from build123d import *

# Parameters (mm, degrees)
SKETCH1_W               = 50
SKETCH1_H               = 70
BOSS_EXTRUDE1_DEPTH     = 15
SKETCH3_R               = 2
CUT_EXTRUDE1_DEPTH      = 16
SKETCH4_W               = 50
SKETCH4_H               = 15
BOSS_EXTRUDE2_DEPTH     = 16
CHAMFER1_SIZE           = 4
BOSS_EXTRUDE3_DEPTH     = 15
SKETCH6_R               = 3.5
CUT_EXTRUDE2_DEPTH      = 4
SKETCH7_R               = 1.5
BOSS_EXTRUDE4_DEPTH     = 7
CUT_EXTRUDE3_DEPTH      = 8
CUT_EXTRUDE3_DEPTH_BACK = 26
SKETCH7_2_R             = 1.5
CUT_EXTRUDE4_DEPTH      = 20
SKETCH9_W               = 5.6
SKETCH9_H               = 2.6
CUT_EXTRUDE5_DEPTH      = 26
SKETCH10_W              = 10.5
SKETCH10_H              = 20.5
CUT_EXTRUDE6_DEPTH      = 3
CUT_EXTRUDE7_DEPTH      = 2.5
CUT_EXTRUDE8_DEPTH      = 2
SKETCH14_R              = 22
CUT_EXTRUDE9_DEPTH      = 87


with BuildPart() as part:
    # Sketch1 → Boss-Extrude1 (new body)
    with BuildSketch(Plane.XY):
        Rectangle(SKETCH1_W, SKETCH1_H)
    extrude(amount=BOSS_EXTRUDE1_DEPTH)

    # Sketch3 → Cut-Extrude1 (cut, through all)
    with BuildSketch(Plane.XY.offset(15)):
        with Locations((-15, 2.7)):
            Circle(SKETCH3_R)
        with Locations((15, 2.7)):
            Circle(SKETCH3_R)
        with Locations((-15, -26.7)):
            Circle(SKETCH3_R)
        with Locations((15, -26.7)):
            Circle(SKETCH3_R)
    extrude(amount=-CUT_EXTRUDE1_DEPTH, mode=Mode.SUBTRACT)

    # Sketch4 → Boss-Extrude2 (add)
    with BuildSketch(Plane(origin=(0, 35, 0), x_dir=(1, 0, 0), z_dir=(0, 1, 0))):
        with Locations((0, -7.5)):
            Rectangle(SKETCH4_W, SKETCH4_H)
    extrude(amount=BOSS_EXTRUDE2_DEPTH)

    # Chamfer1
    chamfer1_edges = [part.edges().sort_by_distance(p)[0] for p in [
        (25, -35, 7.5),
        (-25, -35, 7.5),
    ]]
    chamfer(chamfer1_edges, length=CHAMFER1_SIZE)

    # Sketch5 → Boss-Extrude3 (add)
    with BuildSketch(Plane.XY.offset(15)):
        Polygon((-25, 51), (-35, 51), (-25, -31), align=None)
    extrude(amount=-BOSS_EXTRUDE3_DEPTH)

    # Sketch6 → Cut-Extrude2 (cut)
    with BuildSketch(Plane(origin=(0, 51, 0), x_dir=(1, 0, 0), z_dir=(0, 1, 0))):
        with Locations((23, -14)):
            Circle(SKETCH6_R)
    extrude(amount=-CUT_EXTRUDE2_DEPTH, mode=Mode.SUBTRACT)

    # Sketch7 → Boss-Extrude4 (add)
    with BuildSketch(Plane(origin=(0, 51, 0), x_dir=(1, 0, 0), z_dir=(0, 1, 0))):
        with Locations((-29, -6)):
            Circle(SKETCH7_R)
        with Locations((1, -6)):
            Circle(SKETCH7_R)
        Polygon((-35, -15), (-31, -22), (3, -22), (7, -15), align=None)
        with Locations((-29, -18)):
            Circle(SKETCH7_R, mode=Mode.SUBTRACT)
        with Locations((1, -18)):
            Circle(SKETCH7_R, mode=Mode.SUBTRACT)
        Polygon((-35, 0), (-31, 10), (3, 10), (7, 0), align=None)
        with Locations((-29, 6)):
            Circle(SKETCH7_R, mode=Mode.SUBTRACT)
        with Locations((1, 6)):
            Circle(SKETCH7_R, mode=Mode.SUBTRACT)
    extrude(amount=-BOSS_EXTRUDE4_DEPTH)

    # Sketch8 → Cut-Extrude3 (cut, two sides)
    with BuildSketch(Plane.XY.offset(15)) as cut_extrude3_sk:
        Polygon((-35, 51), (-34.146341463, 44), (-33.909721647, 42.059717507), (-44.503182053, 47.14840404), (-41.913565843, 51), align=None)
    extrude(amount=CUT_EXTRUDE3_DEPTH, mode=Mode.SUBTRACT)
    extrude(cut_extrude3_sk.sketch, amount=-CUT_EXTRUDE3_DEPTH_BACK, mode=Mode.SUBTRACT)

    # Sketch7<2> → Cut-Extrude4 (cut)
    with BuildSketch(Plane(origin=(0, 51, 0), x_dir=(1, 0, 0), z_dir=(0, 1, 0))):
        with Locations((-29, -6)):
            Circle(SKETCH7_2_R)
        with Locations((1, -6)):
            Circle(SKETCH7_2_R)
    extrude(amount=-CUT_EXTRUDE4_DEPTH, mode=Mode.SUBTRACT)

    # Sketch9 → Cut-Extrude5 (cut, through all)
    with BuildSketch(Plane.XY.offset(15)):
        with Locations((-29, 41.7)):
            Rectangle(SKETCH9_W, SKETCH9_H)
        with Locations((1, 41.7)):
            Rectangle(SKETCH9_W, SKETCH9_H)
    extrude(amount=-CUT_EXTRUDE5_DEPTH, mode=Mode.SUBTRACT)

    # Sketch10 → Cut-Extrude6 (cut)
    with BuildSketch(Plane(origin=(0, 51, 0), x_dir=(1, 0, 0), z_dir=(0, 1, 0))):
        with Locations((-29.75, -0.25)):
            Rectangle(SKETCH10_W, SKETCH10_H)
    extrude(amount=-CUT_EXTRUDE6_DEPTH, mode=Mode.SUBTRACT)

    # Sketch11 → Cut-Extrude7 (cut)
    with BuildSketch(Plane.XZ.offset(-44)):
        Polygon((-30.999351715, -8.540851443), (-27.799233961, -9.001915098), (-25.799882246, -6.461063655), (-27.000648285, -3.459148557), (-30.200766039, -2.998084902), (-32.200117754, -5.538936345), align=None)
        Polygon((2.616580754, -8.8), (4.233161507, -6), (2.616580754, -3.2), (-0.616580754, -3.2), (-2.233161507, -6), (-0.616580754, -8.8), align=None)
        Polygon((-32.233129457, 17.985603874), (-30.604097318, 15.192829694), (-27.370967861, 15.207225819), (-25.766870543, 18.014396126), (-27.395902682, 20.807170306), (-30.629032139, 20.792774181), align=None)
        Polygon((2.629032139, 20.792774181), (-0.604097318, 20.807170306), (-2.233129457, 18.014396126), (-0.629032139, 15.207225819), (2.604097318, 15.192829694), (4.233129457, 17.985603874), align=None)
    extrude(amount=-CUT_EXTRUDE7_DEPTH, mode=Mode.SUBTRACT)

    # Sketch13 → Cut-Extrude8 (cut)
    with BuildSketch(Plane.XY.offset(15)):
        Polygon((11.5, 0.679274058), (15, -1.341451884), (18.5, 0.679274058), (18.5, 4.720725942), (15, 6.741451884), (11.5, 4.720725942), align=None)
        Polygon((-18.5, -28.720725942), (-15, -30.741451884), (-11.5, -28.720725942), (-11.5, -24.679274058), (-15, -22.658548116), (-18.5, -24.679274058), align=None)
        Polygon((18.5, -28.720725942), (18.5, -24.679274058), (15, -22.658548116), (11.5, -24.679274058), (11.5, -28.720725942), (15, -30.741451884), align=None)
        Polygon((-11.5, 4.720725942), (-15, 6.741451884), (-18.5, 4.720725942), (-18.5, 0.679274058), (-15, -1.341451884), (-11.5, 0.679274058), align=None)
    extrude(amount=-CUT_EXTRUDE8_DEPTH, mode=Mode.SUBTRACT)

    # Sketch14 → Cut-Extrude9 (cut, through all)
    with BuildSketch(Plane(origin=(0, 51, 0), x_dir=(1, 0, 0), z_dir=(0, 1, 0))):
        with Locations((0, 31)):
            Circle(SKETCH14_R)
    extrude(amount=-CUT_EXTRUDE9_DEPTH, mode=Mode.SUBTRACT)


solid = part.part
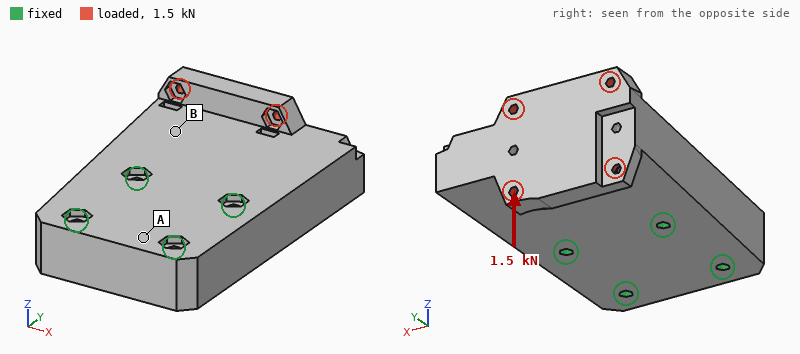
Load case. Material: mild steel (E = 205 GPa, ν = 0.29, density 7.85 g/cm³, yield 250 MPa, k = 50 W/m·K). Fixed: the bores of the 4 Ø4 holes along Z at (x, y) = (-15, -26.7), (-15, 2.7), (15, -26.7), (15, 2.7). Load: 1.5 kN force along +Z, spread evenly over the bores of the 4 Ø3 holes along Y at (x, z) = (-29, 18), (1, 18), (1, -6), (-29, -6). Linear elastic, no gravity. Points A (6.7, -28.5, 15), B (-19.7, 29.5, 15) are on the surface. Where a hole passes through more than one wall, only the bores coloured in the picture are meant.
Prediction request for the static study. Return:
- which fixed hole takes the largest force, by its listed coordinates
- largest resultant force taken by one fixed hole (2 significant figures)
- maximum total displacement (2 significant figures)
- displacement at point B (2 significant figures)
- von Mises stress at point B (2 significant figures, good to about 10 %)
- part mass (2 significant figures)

(-15, 2.7)
1.8 kN
29 µm
12 µm
14 MPa
570 g
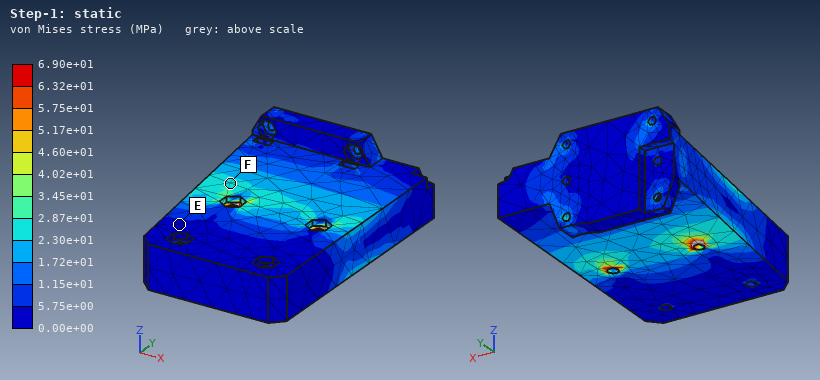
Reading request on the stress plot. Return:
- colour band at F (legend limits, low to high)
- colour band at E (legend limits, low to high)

2.30e+01 to 2.87e+01 MPa
0.00e+00 to 5.75e+00 MPa
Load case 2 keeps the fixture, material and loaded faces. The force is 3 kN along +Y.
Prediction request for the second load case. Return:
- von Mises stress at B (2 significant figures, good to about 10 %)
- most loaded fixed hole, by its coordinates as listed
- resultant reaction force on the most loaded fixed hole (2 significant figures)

7.0 MPa
(-15, 2.7)
1.9 kN
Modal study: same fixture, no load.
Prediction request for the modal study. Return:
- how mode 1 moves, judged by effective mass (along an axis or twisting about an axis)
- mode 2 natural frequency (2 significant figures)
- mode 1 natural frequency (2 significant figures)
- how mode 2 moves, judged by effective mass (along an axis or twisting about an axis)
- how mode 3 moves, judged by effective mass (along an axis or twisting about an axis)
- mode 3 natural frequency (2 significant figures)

along Z
7600 Hz
3700 Hz
twisting about Y
along X
8700 Hz
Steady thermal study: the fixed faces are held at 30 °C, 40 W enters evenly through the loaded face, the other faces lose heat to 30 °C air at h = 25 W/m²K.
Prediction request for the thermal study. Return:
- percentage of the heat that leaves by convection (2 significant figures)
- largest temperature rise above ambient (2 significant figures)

20 %
75 K
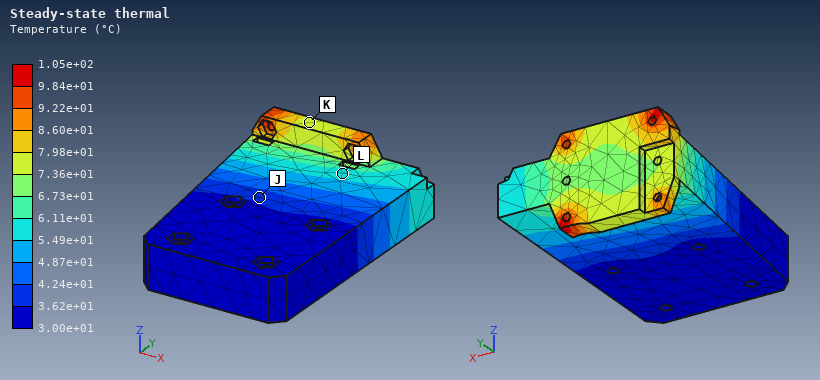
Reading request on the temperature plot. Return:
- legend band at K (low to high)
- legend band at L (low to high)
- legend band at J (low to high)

7.36e+01 to 7.98e+01 °C
5.49e+01 to 6.11e+01 °C
3.62e+01 to 4.24e+01 °C
